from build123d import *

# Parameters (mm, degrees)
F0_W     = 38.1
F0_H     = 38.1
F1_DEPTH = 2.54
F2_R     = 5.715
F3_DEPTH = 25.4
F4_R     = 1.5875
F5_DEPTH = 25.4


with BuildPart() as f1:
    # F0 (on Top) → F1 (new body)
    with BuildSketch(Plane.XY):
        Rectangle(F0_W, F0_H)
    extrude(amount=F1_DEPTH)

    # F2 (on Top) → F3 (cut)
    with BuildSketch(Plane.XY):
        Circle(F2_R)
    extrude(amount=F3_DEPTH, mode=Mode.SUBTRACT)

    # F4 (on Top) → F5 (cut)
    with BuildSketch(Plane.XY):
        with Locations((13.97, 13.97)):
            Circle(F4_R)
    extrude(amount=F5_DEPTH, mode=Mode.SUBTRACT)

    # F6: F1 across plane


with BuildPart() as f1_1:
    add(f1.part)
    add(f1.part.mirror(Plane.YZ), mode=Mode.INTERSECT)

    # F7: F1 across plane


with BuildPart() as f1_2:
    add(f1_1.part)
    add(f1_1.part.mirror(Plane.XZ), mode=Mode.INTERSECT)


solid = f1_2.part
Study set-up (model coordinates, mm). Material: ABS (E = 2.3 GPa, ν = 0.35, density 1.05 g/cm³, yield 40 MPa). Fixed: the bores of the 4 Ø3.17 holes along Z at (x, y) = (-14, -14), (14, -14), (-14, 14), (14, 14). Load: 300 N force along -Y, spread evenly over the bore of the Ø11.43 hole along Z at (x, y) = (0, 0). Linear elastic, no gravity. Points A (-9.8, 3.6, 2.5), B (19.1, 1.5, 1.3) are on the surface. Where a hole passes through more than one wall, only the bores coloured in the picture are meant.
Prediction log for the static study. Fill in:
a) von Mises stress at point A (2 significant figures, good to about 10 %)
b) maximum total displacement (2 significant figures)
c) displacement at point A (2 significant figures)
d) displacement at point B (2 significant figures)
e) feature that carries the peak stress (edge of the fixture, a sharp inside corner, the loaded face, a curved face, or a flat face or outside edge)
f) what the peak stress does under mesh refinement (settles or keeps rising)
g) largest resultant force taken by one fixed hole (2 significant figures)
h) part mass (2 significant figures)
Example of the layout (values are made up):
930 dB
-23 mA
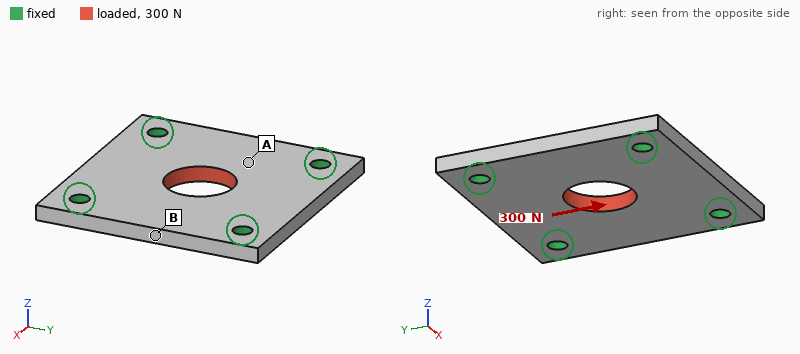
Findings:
2.8 MPa
31 µm
14 µm
4.8 µm
edge of the fixture
keeps rising
82 N
3.5 g
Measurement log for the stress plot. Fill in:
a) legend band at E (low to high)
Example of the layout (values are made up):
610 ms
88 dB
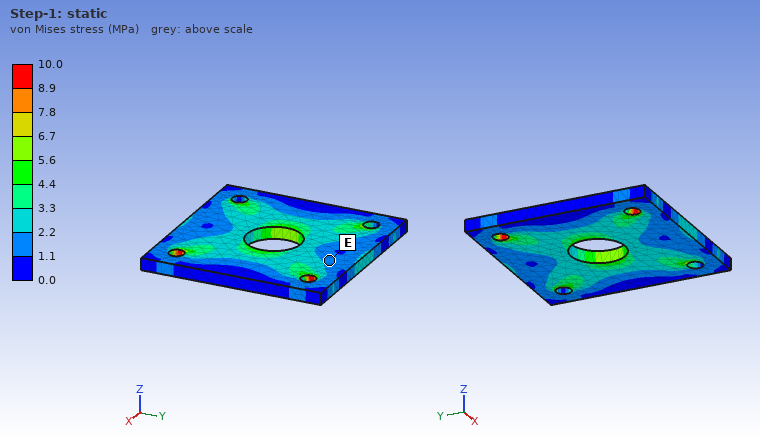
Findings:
1.1 to 2.2 MPa
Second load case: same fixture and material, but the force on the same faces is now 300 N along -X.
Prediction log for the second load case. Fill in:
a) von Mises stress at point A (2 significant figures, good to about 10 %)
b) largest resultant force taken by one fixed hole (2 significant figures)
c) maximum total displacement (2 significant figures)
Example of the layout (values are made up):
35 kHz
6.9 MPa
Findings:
2.5 MPa
82 N
31 µm
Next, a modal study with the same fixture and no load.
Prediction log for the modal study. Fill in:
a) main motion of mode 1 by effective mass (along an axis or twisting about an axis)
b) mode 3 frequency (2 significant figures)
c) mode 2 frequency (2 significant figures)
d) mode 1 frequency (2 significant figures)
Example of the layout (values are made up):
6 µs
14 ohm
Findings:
along Z
5400 Hz
5400 Hz
3900 Hz
